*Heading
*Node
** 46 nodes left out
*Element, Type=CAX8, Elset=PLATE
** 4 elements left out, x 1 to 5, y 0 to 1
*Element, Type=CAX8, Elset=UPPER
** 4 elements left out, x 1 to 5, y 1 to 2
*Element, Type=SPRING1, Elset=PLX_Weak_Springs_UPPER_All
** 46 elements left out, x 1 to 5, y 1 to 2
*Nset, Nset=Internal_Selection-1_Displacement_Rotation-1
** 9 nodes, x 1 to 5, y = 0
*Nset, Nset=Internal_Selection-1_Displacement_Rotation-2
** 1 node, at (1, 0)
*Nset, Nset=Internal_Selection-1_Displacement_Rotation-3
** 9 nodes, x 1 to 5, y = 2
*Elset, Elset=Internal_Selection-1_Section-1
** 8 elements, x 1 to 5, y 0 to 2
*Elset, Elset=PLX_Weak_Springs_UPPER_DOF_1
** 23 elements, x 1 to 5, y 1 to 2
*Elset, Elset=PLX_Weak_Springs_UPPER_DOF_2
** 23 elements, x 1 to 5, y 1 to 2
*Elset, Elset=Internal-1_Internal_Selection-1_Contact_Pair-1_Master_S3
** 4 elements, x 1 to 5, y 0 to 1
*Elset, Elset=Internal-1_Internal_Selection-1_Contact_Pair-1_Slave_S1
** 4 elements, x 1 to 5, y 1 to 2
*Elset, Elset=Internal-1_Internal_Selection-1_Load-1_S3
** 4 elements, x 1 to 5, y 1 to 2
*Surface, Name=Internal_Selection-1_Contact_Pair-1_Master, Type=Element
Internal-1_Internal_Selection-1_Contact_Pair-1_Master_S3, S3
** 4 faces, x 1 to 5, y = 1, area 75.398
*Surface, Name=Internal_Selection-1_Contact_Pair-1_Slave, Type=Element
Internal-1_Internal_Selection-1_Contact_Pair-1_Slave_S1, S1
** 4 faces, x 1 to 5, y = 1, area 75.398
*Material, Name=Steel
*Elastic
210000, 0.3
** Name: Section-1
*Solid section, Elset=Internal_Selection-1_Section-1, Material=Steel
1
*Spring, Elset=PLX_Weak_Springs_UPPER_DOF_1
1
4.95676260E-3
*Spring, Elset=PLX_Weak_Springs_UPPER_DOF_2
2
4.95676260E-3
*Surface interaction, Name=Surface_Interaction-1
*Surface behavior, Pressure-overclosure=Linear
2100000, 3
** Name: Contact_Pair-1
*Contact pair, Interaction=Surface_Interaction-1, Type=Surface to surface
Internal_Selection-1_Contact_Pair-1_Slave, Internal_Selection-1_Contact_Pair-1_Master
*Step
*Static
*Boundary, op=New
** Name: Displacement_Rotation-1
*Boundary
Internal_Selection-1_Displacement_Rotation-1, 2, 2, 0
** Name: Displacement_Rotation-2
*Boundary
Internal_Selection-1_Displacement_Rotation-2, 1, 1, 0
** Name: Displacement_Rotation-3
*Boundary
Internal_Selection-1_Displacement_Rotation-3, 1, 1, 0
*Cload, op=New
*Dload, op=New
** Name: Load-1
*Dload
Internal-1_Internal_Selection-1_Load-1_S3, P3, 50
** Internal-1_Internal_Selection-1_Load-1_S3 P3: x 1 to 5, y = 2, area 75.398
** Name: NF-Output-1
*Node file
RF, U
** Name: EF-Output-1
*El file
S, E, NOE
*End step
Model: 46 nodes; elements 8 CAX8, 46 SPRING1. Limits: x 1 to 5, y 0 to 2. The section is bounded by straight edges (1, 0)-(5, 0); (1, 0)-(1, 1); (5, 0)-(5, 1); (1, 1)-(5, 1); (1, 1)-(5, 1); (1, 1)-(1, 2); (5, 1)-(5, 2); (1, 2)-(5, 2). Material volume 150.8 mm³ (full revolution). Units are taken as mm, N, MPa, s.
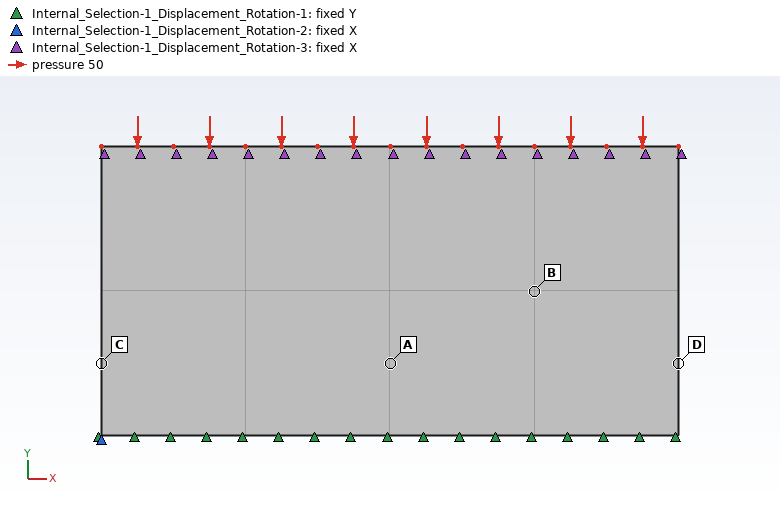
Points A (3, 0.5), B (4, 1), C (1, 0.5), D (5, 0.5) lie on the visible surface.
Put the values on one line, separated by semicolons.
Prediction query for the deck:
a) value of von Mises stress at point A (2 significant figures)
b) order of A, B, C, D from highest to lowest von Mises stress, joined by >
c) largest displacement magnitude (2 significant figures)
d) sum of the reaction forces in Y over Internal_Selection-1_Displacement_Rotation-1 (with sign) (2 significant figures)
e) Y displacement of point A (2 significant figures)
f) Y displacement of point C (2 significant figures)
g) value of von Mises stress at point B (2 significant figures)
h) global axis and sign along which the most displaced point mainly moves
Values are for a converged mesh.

54 MPa; A > B > C > D; 4.9e-04 mm; 3800 N; -1.3e-04 mm; -1.1e-04 mm; 48 MPa; -Y
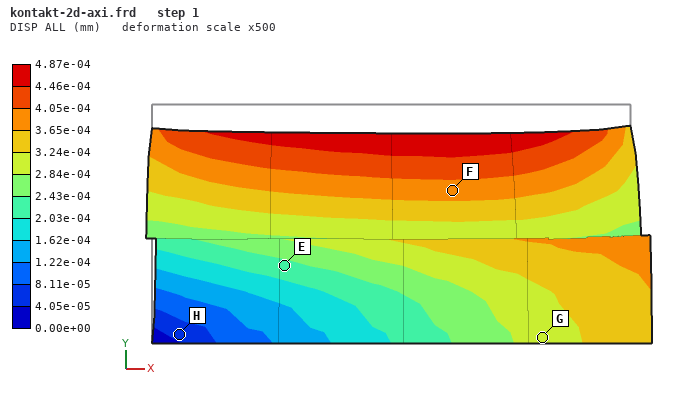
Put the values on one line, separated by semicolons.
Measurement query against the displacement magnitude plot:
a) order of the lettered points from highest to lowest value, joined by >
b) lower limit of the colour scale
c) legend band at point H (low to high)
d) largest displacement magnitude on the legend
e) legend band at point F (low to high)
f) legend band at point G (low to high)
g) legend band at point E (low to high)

F > G > E > H; 0.00e+00 mm; 4.05e-05 to 8.11e-05 mm; 4.87e-04 mm; 3.65e-04 to 4.05e-04 mm; 2.84e-04 to 3.24e-04 mm; 2.03e-04 to 2.43e-04 mm
